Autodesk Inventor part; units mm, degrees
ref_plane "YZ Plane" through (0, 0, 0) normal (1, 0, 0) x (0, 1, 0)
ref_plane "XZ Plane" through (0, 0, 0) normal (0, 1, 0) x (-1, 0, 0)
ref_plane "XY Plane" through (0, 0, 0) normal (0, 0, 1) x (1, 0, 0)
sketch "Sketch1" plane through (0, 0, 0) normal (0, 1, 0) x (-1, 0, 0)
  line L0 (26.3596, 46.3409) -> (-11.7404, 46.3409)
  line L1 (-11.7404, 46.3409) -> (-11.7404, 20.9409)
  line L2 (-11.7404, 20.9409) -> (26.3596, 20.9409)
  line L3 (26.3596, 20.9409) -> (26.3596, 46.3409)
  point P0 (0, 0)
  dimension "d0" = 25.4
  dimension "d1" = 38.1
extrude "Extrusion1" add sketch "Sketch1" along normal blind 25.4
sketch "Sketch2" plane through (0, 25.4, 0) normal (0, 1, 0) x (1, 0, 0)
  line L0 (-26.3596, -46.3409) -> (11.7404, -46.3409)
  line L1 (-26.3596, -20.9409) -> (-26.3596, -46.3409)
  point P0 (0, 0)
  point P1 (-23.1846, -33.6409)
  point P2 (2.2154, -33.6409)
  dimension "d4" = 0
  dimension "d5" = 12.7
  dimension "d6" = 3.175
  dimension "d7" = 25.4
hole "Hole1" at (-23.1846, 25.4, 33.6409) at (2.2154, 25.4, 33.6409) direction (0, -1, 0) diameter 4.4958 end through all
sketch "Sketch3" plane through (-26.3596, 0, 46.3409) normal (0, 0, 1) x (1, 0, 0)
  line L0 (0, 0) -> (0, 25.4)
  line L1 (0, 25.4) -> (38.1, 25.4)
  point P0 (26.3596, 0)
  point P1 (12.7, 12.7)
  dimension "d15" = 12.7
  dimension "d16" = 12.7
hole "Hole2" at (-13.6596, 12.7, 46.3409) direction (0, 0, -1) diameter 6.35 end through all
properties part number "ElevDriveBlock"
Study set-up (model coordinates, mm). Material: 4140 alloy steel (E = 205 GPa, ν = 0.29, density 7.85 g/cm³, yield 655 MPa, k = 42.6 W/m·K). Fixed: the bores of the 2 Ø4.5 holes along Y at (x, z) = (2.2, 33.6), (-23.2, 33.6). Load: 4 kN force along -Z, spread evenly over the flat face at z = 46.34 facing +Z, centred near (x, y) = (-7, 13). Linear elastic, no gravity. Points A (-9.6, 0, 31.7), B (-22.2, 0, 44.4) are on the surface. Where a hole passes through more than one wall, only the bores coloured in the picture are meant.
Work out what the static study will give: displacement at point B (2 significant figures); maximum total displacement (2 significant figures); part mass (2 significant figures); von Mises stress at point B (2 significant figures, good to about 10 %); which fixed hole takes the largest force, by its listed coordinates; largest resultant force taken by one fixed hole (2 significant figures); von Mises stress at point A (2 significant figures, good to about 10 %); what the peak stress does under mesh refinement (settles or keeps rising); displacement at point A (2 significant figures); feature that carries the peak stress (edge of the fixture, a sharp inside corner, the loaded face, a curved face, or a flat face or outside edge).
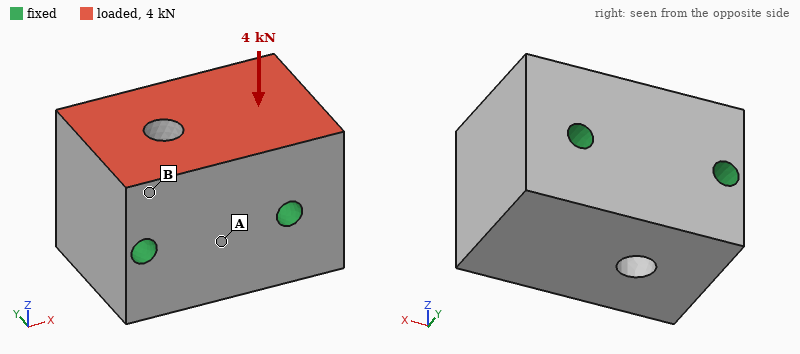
0.27 µm
0.45 µm
180 g
4.3 MPa
(2.2, 33.6)
2.5 kN
1.9 MPa
keeps rising
0.24 µm
edge of the fixture
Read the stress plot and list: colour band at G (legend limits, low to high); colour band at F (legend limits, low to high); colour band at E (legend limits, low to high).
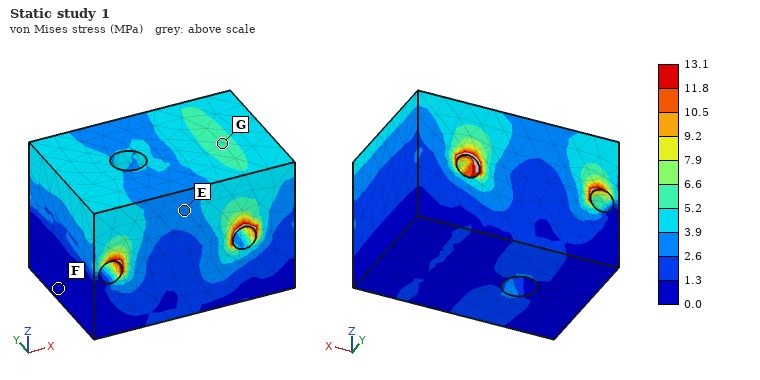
5.2 to 6.6 MPa
0.0 to 1.3 MPa
2.6 to 3.9 MPa
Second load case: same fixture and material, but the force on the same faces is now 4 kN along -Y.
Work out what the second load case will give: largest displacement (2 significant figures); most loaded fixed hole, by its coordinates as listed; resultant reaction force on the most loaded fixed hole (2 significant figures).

1.8 µm
(2.2, 33.6)
2.4 kN
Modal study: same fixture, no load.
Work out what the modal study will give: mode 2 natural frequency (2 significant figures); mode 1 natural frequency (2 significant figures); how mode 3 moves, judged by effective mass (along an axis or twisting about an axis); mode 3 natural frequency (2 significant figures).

42 kHz
42 kHz
along Y
44 kHz
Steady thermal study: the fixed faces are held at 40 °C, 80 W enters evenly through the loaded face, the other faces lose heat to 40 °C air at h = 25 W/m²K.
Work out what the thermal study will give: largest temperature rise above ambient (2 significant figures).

29 K
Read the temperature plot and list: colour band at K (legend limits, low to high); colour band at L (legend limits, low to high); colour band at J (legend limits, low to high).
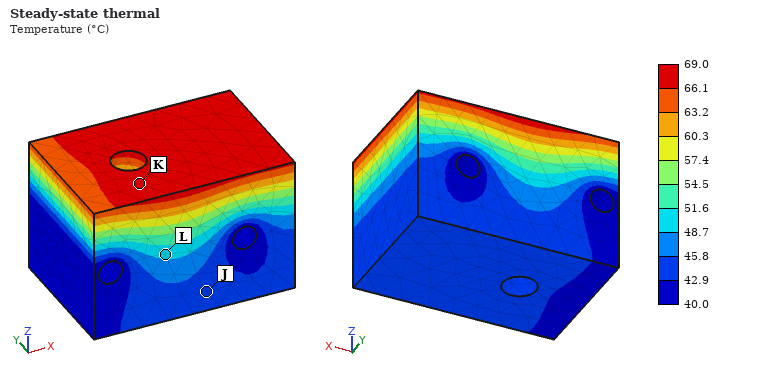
66.1 to 69.0 °C
48.7 to 51.6 °C
42.9 to 45.8 °C
